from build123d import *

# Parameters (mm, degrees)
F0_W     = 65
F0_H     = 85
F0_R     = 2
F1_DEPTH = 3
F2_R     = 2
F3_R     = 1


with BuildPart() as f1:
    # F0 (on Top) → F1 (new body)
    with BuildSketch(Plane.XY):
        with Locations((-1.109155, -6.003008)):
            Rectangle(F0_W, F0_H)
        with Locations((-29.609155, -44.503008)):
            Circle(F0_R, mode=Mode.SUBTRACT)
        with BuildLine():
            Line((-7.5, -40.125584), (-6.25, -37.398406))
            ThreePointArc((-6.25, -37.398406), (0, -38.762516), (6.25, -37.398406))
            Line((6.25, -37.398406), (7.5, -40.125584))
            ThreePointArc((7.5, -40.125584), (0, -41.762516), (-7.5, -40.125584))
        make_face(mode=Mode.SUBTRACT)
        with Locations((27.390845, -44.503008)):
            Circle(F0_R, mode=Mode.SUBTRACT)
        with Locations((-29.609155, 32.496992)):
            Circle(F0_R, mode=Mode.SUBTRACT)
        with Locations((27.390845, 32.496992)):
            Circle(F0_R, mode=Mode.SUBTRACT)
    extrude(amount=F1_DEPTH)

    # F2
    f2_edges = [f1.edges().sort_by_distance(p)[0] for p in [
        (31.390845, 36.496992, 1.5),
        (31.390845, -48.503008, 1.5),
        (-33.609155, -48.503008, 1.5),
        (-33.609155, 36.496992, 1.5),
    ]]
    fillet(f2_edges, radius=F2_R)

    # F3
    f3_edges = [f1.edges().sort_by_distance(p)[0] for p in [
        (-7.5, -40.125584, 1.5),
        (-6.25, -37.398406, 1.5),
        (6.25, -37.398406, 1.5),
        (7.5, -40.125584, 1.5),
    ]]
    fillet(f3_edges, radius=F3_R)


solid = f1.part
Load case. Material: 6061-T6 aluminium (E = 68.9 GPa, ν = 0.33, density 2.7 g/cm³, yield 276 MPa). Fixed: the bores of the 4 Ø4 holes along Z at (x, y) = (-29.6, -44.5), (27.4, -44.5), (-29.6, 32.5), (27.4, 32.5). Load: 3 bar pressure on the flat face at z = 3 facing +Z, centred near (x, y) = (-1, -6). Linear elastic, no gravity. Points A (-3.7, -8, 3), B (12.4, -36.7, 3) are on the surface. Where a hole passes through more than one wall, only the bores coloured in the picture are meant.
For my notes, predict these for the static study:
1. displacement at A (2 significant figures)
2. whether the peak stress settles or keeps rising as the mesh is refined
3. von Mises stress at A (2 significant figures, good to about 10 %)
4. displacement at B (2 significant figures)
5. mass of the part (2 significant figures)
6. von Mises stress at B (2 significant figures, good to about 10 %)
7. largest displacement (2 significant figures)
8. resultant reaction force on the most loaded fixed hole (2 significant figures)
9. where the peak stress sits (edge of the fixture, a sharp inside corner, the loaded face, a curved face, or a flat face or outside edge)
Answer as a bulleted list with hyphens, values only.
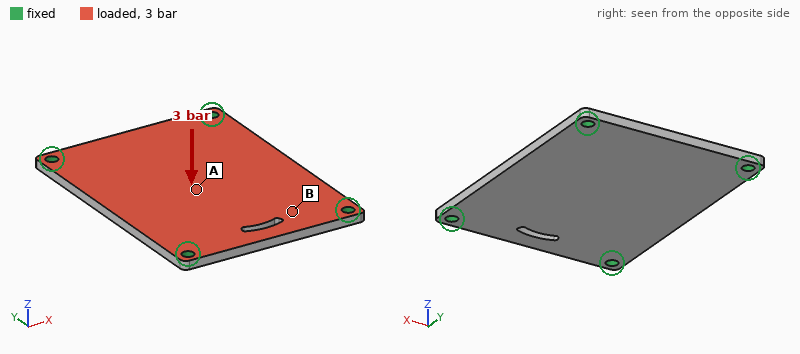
- 0.30 mm
- keeps rising
- 54 MPa
- 0.11 mm
- 44 g
- 22 MPa
- 0.31 mm
- 410 N
- edge of the fixture
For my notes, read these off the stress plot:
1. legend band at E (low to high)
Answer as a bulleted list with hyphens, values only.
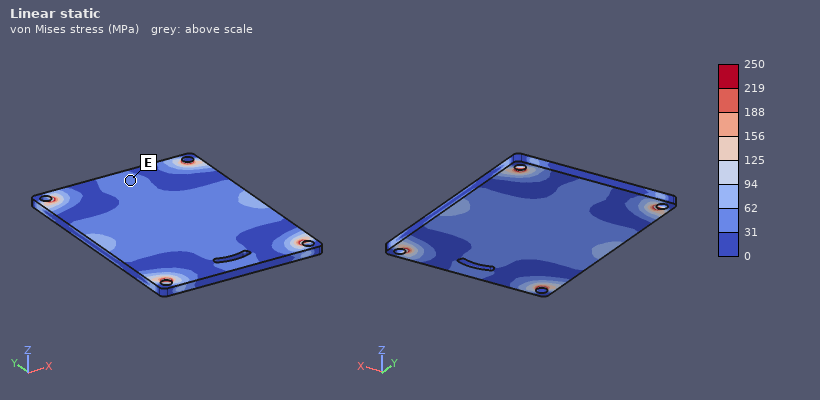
- 31 to 62 MPa
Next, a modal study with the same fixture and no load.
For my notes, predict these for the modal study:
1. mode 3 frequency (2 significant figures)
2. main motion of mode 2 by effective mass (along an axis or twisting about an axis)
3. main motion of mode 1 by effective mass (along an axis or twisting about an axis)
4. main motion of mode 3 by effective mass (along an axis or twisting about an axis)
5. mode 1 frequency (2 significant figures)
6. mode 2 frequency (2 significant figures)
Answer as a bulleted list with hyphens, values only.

- 4600 Hz
- twisting about Y
- along Z
- twisting about X
- 2100 Hz
- 3300 Hz
